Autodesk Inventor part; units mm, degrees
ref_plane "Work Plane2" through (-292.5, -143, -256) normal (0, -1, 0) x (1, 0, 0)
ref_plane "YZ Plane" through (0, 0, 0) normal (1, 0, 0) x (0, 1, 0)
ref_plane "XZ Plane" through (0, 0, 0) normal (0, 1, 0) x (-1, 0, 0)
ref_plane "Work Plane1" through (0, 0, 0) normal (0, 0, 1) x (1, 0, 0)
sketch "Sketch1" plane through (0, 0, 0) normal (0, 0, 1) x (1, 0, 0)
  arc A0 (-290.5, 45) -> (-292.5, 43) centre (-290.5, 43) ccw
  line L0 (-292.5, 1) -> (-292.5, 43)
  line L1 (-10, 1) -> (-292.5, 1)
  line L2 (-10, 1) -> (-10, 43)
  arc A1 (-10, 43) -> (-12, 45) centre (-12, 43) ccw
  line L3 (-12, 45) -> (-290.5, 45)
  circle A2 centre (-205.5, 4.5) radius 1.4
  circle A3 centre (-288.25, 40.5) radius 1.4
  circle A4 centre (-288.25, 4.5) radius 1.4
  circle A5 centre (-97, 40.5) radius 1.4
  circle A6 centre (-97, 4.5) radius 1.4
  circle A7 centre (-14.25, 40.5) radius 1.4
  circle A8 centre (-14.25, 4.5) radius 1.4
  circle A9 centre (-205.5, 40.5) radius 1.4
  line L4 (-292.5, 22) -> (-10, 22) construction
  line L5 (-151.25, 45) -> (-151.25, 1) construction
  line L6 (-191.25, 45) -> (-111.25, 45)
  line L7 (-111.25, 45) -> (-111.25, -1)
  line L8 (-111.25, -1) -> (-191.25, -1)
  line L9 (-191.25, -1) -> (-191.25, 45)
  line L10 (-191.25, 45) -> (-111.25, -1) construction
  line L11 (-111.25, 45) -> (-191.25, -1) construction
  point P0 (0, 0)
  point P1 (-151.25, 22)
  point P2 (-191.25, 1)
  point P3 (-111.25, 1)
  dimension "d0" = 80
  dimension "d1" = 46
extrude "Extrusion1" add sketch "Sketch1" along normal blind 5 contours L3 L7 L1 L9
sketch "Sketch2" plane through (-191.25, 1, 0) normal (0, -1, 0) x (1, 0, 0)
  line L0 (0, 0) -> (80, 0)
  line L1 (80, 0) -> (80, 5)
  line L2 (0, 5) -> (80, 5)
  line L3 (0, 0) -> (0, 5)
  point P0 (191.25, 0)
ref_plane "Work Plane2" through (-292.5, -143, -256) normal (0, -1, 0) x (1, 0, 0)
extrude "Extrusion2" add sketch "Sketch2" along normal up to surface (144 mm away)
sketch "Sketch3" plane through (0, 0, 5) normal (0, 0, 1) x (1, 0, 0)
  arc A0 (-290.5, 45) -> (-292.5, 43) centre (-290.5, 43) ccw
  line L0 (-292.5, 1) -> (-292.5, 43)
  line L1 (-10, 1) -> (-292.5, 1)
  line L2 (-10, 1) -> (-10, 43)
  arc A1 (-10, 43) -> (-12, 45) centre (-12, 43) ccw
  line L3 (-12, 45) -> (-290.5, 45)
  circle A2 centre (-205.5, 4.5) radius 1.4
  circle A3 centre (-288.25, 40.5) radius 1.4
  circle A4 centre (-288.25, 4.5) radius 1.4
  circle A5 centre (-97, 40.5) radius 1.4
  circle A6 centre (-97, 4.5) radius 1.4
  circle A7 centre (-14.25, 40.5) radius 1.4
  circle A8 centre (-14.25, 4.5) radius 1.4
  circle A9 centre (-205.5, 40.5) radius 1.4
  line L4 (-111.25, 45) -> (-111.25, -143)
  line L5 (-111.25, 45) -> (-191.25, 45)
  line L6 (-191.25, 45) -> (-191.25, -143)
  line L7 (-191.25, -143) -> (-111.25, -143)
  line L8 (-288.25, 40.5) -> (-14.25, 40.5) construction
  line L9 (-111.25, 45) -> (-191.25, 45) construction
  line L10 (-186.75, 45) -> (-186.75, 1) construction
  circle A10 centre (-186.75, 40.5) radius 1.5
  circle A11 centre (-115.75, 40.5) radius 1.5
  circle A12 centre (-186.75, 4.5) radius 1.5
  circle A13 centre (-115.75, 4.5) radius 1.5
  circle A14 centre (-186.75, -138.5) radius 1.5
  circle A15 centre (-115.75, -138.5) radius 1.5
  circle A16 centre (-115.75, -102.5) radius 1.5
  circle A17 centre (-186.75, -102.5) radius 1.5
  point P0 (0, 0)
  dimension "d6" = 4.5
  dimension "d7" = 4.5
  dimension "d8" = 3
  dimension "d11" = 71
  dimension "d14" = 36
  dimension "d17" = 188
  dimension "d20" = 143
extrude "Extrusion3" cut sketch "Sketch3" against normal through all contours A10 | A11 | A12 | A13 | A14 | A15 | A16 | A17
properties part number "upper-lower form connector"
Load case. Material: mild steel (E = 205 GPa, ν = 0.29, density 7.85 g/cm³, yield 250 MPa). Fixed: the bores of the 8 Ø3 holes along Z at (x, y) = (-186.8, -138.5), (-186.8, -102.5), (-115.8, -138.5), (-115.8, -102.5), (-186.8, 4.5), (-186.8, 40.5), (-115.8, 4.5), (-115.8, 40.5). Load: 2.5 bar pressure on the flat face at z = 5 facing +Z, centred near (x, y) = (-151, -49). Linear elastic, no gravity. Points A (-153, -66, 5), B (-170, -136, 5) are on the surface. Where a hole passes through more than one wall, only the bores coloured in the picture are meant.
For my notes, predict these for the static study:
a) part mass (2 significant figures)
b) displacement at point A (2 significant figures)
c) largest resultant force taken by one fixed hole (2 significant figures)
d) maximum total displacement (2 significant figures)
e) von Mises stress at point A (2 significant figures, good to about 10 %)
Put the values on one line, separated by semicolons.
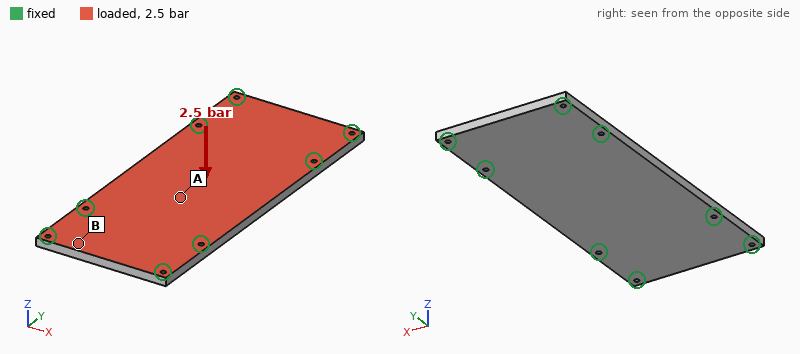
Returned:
590 g; 58 µm; 810 N; 66 µm; 22 MPa
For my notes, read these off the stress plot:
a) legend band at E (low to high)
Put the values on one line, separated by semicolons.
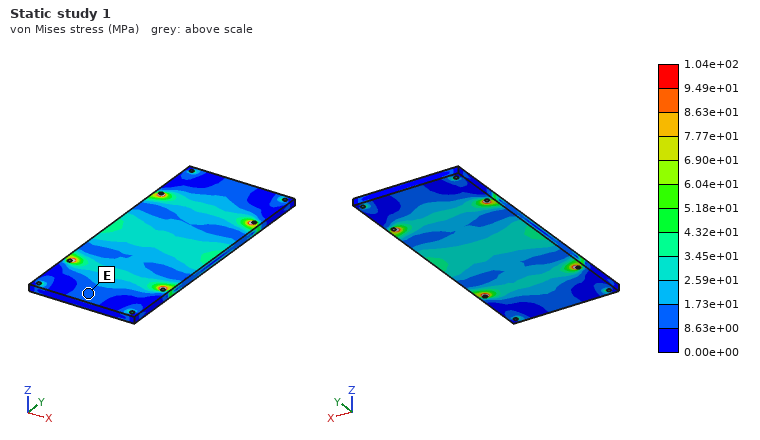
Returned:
8.63e+00 to 1.73e+01 MPa
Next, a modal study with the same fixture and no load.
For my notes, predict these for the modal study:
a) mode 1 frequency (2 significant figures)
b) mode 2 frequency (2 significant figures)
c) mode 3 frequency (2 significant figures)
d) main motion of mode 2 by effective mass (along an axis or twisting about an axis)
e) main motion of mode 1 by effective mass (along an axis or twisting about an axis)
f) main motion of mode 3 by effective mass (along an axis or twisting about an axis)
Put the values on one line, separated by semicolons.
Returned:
1800 Hz; 2900 Hz; 4100 Hz; twisting about Y; along Z; twisting about X
